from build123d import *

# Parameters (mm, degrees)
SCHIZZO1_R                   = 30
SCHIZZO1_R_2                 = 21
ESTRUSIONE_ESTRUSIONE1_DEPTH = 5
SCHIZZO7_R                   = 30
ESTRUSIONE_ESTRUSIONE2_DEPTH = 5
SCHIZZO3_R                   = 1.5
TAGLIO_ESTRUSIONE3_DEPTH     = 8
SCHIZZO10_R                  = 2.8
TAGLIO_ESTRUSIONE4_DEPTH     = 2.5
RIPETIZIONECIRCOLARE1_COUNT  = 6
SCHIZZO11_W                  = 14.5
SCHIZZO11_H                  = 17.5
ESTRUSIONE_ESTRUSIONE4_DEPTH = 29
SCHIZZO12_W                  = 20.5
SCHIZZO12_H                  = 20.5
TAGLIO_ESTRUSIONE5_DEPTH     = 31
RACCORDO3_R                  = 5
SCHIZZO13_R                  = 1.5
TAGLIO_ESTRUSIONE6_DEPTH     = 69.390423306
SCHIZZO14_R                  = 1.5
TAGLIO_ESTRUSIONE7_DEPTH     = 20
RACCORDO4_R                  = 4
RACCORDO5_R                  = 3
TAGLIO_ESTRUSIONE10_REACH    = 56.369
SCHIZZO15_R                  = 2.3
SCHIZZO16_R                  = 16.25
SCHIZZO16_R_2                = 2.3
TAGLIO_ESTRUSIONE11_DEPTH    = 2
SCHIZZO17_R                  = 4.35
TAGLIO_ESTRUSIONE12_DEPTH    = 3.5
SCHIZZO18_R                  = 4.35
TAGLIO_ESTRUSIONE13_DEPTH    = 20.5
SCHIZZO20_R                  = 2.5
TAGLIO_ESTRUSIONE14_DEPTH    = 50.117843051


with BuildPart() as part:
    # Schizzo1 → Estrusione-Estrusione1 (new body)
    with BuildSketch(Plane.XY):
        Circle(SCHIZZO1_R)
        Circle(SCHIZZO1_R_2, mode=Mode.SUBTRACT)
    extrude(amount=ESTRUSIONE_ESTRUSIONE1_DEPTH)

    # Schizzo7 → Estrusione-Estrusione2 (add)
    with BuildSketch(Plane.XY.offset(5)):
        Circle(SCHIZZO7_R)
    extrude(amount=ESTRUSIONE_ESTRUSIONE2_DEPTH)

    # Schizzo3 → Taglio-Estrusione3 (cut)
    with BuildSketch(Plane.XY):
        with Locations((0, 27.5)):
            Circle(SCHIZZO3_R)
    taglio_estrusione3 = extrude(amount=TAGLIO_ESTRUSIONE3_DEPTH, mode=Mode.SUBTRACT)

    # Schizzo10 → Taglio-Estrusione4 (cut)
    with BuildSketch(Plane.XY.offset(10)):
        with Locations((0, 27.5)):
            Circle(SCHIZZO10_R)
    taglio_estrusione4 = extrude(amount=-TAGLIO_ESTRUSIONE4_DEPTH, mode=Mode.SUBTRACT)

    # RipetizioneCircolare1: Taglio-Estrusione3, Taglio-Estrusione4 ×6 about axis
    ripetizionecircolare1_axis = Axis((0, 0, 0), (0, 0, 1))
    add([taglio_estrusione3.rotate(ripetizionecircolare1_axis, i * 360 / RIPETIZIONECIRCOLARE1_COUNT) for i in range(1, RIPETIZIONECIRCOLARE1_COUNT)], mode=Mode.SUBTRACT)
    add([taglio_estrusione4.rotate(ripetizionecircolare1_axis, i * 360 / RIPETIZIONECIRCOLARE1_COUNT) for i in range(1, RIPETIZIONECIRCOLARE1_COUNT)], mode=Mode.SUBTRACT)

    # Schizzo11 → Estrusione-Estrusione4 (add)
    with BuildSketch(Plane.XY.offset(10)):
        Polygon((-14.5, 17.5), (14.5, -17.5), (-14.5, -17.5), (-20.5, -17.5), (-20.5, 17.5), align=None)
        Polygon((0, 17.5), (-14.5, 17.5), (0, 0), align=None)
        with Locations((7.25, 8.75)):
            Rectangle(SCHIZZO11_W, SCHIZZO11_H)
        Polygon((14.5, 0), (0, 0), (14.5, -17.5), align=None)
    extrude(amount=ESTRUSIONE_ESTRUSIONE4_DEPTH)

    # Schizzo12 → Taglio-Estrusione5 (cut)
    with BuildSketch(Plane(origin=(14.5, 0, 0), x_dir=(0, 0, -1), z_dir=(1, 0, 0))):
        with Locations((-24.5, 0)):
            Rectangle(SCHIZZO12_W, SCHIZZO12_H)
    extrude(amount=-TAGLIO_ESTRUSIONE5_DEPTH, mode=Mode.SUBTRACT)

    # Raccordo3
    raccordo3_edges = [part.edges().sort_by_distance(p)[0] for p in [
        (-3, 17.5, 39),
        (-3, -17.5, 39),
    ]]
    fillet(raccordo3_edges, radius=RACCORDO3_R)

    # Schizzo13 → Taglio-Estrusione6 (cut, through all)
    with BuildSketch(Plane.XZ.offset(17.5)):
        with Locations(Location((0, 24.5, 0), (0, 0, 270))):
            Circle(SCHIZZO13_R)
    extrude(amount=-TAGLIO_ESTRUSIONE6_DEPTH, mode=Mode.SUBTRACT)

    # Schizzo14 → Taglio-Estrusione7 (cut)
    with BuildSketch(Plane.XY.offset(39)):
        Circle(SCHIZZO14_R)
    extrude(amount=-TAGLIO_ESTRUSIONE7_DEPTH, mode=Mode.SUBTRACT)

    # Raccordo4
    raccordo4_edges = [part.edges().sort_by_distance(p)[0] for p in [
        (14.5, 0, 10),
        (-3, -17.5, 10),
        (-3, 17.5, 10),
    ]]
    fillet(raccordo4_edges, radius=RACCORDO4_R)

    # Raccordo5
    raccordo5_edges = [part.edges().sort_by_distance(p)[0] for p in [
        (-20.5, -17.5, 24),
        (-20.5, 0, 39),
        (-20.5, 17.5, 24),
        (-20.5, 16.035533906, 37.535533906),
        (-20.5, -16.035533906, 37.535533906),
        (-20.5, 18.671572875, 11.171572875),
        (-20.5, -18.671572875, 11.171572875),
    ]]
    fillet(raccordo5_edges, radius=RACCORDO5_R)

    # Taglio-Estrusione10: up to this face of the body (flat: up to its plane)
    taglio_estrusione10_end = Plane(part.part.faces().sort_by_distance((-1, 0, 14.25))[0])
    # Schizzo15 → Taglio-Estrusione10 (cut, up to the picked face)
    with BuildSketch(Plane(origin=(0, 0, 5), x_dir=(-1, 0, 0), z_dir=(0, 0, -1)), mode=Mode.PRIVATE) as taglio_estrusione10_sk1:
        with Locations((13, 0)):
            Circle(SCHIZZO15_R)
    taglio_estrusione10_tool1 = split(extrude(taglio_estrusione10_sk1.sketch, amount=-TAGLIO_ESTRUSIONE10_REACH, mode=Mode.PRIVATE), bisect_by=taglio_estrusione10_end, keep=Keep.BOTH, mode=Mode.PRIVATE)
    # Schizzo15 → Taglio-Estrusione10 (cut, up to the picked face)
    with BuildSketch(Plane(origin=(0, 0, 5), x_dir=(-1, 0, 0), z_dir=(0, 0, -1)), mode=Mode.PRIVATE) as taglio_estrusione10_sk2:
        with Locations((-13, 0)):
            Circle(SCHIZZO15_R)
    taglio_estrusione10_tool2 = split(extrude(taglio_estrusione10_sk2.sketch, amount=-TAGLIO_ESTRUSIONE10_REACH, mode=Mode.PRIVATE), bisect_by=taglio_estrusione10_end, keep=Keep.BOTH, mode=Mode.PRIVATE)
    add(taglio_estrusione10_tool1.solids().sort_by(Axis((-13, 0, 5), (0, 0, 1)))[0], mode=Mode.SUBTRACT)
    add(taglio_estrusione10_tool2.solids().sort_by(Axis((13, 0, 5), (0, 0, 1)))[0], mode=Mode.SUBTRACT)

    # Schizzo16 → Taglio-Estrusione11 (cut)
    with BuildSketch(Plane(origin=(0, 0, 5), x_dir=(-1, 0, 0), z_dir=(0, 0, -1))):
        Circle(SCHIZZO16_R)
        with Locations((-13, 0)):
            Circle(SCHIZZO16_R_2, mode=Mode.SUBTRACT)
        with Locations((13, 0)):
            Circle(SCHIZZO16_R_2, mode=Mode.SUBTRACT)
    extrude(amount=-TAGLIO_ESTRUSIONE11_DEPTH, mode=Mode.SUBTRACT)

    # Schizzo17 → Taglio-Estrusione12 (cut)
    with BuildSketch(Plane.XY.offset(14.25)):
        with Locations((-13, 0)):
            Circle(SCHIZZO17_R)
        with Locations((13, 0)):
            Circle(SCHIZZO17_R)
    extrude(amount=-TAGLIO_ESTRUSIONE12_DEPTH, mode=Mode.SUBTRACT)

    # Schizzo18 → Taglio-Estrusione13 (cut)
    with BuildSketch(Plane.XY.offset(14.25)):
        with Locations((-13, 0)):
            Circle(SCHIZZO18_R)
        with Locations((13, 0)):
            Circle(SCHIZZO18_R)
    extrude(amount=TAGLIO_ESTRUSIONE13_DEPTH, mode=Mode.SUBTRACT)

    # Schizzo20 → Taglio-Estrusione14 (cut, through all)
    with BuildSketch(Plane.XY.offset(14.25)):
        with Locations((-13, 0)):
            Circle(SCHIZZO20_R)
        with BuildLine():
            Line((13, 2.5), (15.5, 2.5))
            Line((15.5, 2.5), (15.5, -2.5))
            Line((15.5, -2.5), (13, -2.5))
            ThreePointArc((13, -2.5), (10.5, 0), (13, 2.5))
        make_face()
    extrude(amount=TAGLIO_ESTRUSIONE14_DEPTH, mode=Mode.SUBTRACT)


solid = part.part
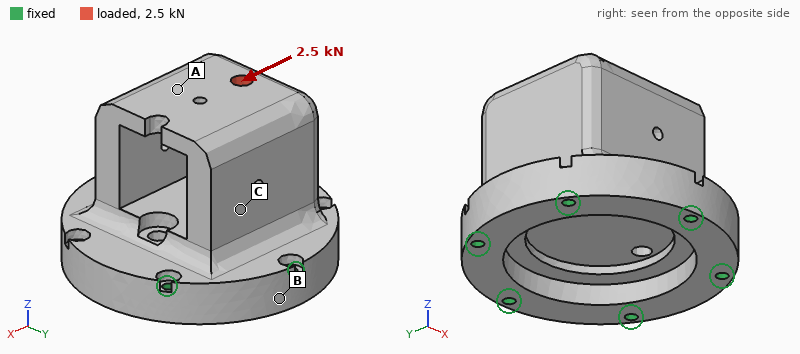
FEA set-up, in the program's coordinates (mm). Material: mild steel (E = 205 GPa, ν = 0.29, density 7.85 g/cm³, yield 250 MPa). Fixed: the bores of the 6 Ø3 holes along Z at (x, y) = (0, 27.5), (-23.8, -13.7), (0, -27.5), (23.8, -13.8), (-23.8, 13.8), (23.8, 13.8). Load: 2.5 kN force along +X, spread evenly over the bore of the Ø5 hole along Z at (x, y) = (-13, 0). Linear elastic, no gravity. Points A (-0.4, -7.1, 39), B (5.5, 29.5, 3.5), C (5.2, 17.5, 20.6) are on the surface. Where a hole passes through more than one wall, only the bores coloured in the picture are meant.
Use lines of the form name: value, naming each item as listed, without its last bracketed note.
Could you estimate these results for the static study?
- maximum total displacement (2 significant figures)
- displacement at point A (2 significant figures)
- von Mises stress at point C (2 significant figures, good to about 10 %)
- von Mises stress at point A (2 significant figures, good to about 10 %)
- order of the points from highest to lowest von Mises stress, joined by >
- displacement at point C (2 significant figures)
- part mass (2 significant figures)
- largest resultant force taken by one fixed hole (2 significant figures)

maximum total displacement: 9.1 µm
displacement at point A: 6.2 µm
von Mises stress at point C: 10 MPa
von Mises stress at point A: 16 MPa
order of the points from highest to lowest von Mises stress, joined by >: A > C > B
displacement at point C: 2.3 µm
part mass: 320 g
largest resultant force taken by one fixed hole: 1.2 kN
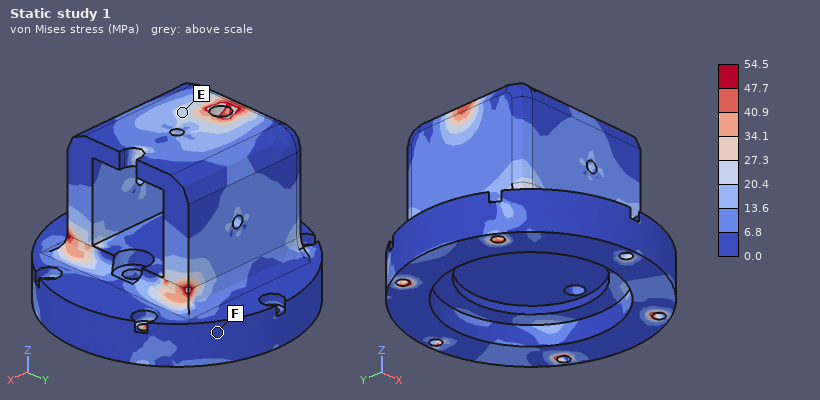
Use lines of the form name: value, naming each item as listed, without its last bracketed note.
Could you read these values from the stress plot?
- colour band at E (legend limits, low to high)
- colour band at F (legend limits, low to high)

colour band at E: 20.4 to 27.3 MPa
colour band at F: 0.0 to 6.8 MPa
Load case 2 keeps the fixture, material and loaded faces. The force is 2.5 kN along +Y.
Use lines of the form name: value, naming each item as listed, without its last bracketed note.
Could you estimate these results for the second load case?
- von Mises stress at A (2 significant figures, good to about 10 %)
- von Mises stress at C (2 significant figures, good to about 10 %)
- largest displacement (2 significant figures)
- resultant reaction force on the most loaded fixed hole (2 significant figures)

von Mises stress at A: 20 MPa
von Mises stress at C: 16 MPa
largest displacement: 11 µm
resultant reaction force on the most loaded fixed hole: 1.2 kN
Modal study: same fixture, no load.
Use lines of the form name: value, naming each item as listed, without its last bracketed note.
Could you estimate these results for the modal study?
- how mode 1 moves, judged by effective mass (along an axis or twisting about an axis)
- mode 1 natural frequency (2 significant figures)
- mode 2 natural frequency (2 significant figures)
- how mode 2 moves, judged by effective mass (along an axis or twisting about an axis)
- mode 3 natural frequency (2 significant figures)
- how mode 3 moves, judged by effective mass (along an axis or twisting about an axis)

how mode 1 moves, judged by effective mass: along Y
mode 1 natural frequency: 8800 Hz
mode 2 natural frequency: 12 kHz
how mode 2 moves, judged by effective mass: along X
mode 3 natural frequency: 17 kHz
how mode 3 moves, judged by effective mass: along Z
